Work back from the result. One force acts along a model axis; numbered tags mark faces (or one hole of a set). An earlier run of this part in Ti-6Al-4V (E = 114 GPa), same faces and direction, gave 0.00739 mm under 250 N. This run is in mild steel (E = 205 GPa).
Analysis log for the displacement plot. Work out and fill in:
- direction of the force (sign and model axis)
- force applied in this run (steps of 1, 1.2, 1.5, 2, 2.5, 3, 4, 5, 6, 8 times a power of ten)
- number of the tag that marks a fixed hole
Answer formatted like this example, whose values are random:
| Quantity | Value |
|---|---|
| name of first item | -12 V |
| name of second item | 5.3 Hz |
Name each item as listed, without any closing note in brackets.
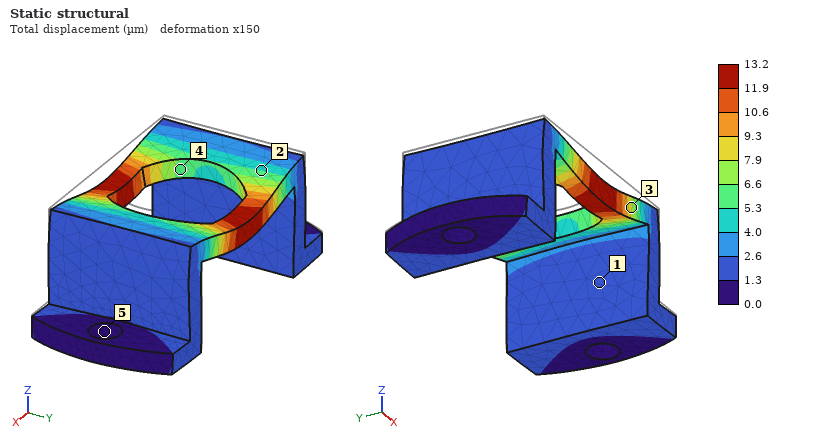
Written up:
| Quantity | Value |
|---|---|
| direction of the force | -Z |
| force applied in this run | 800 N |
| number of the tag that marks a fixed hole | 5 |
